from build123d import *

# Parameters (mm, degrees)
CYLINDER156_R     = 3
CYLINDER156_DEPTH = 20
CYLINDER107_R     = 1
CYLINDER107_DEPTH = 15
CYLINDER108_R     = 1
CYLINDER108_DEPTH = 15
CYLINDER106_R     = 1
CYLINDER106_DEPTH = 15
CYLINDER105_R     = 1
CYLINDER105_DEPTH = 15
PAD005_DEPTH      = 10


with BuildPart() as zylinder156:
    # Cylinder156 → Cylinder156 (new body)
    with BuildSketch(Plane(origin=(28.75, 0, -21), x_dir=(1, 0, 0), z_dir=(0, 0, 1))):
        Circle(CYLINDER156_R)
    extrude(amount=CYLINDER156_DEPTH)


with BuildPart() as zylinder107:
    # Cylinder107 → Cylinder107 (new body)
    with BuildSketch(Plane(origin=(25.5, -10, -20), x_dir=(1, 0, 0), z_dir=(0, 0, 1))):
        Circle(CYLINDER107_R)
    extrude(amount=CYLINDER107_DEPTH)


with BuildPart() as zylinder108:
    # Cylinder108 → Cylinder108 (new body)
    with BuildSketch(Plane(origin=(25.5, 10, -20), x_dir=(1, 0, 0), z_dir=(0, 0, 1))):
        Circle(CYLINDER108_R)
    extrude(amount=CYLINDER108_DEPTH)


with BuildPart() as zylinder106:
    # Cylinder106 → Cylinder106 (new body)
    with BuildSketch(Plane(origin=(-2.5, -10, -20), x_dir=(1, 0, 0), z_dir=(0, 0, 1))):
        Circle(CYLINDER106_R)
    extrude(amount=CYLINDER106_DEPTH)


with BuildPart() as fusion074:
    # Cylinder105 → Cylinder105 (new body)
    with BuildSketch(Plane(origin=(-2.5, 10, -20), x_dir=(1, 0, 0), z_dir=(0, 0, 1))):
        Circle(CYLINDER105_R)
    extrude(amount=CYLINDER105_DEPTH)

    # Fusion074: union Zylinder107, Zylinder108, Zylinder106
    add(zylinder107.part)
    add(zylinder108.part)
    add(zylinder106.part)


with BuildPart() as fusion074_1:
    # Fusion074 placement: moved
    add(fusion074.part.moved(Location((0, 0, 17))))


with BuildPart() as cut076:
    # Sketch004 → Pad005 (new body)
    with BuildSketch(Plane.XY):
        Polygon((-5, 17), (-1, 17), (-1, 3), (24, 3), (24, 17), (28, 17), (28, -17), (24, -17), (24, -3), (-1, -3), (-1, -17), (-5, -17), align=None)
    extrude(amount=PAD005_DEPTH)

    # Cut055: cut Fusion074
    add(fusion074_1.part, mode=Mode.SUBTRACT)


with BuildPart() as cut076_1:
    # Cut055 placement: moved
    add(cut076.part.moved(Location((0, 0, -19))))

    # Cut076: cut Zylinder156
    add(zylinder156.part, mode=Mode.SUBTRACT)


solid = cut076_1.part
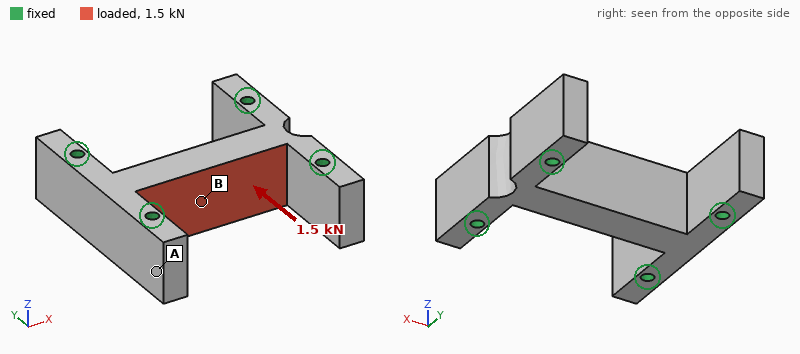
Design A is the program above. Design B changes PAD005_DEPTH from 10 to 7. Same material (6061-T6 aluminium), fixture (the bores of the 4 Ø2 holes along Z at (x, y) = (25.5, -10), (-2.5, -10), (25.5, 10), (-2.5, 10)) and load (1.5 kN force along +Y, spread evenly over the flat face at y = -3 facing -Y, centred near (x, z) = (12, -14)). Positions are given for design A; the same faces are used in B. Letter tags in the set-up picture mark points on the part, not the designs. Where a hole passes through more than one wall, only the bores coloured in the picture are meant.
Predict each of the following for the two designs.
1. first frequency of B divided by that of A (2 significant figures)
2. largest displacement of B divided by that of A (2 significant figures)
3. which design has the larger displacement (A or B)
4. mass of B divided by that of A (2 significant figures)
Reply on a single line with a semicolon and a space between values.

0.82; 1.4; B; 0.70
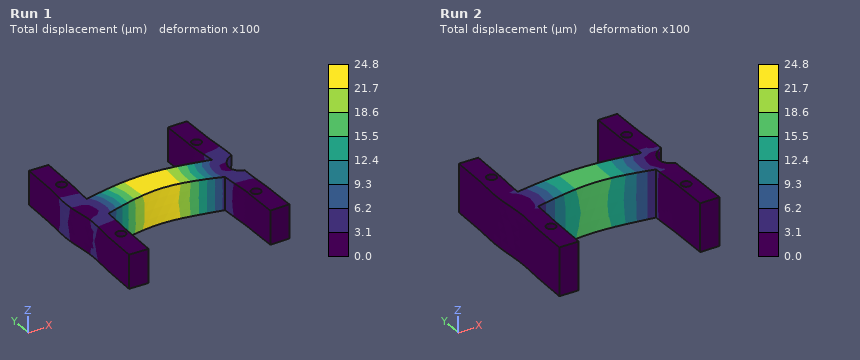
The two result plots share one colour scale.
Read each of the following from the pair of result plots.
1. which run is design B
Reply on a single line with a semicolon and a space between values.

Run 1
